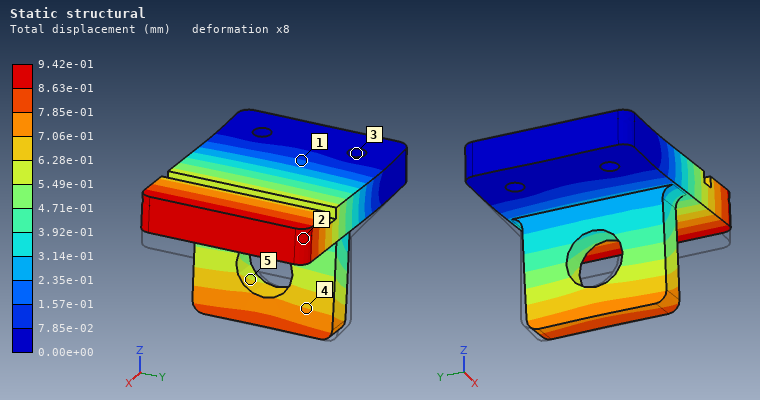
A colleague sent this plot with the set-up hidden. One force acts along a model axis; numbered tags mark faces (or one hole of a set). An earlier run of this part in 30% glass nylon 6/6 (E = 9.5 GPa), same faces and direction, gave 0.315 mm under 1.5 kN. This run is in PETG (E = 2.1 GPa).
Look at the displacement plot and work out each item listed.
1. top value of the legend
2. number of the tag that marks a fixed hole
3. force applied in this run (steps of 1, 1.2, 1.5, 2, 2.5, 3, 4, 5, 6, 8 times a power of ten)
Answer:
9.42e-01 mm
3
1 kN
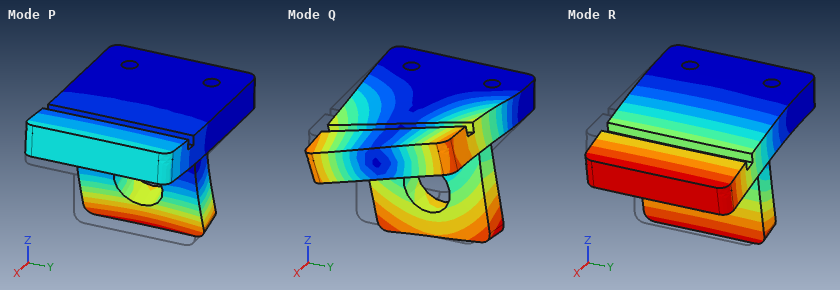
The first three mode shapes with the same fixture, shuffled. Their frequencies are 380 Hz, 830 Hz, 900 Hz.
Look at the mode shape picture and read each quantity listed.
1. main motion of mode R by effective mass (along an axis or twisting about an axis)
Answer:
along Z
